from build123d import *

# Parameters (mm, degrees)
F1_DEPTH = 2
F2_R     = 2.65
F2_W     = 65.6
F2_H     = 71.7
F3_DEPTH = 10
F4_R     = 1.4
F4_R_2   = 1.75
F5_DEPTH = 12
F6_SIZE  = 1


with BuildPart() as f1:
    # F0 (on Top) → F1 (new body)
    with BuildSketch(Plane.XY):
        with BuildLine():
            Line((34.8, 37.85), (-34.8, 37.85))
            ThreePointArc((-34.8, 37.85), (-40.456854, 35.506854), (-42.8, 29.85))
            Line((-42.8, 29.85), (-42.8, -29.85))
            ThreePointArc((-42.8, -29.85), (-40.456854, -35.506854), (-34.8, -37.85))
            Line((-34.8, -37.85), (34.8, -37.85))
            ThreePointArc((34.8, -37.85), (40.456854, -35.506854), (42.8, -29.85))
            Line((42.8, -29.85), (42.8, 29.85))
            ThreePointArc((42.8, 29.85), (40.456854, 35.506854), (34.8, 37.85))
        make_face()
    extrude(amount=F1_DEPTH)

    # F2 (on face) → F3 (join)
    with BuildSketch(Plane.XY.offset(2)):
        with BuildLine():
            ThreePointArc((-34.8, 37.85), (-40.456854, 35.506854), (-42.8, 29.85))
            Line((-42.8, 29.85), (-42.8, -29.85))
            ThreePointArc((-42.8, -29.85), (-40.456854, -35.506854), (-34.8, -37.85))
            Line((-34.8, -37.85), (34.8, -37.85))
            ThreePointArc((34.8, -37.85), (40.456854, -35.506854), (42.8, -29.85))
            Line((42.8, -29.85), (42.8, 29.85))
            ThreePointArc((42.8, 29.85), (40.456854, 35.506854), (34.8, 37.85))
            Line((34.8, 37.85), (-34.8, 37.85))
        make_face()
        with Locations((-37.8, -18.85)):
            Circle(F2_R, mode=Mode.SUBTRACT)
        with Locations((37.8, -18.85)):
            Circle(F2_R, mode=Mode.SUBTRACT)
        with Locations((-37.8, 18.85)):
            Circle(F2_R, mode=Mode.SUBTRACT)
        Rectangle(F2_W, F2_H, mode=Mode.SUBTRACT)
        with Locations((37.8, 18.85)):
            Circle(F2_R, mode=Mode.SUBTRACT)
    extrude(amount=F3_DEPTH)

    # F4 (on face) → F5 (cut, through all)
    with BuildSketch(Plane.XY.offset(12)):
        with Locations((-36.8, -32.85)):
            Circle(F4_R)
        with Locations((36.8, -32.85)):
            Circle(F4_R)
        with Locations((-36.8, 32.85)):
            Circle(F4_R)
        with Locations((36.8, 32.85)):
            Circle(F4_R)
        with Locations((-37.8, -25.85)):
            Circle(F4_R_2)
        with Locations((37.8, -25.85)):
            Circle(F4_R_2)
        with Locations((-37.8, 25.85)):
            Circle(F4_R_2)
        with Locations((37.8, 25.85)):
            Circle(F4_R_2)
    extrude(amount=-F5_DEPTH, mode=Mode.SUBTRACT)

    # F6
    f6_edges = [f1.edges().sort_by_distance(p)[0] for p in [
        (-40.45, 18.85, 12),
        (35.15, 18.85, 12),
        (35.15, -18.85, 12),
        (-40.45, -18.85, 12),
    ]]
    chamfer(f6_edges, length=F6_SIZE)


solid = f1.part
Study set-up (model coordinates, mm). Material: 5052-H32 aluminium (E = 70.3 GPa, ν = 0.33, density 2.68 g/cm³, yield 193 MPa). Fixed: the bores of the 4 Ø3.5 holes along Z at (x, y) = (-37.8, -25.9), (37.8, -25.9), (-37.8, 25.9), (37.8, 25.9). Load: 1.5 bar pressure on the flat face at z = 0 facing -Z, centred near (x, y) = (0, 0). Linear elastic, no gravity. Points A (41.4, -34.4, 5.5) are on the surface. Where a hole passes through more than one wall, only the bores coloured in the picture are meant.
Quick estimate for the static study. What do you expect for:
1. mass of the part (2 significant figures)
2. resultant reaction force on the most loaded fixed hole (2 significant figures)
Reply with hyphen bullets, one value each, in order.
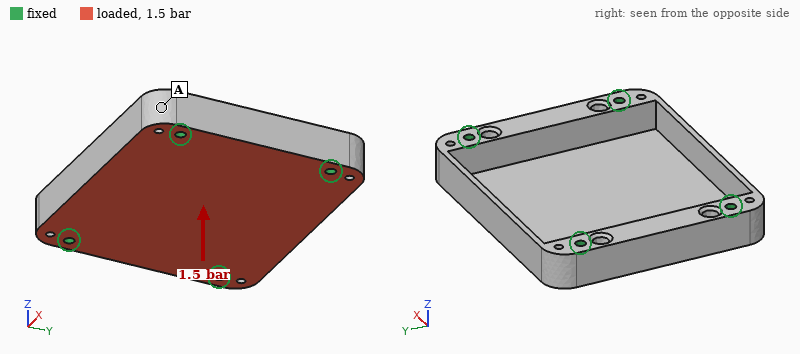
- 76 g
- 250 N
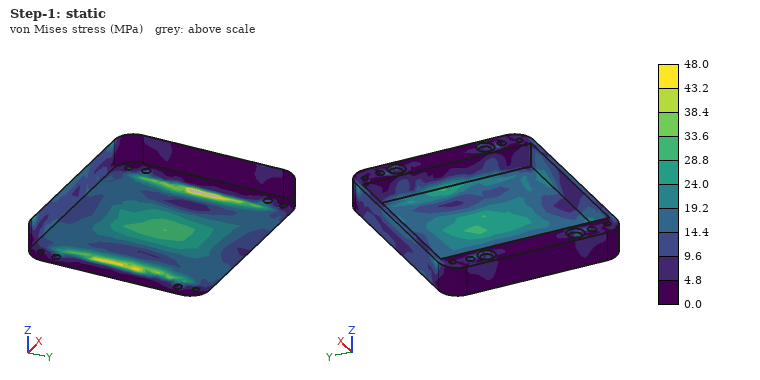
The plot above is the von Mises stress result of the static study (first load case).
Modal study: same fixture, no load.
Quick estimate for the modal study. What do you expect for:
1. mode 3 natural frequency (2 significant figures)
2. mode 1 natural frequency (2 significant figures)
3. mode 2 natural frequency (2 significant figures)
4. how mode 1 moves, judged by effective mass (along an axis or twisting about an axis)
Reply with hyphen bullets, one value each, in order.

- 7200 Hz
- 3000 Hz
- 5000 Hz
- along Z
